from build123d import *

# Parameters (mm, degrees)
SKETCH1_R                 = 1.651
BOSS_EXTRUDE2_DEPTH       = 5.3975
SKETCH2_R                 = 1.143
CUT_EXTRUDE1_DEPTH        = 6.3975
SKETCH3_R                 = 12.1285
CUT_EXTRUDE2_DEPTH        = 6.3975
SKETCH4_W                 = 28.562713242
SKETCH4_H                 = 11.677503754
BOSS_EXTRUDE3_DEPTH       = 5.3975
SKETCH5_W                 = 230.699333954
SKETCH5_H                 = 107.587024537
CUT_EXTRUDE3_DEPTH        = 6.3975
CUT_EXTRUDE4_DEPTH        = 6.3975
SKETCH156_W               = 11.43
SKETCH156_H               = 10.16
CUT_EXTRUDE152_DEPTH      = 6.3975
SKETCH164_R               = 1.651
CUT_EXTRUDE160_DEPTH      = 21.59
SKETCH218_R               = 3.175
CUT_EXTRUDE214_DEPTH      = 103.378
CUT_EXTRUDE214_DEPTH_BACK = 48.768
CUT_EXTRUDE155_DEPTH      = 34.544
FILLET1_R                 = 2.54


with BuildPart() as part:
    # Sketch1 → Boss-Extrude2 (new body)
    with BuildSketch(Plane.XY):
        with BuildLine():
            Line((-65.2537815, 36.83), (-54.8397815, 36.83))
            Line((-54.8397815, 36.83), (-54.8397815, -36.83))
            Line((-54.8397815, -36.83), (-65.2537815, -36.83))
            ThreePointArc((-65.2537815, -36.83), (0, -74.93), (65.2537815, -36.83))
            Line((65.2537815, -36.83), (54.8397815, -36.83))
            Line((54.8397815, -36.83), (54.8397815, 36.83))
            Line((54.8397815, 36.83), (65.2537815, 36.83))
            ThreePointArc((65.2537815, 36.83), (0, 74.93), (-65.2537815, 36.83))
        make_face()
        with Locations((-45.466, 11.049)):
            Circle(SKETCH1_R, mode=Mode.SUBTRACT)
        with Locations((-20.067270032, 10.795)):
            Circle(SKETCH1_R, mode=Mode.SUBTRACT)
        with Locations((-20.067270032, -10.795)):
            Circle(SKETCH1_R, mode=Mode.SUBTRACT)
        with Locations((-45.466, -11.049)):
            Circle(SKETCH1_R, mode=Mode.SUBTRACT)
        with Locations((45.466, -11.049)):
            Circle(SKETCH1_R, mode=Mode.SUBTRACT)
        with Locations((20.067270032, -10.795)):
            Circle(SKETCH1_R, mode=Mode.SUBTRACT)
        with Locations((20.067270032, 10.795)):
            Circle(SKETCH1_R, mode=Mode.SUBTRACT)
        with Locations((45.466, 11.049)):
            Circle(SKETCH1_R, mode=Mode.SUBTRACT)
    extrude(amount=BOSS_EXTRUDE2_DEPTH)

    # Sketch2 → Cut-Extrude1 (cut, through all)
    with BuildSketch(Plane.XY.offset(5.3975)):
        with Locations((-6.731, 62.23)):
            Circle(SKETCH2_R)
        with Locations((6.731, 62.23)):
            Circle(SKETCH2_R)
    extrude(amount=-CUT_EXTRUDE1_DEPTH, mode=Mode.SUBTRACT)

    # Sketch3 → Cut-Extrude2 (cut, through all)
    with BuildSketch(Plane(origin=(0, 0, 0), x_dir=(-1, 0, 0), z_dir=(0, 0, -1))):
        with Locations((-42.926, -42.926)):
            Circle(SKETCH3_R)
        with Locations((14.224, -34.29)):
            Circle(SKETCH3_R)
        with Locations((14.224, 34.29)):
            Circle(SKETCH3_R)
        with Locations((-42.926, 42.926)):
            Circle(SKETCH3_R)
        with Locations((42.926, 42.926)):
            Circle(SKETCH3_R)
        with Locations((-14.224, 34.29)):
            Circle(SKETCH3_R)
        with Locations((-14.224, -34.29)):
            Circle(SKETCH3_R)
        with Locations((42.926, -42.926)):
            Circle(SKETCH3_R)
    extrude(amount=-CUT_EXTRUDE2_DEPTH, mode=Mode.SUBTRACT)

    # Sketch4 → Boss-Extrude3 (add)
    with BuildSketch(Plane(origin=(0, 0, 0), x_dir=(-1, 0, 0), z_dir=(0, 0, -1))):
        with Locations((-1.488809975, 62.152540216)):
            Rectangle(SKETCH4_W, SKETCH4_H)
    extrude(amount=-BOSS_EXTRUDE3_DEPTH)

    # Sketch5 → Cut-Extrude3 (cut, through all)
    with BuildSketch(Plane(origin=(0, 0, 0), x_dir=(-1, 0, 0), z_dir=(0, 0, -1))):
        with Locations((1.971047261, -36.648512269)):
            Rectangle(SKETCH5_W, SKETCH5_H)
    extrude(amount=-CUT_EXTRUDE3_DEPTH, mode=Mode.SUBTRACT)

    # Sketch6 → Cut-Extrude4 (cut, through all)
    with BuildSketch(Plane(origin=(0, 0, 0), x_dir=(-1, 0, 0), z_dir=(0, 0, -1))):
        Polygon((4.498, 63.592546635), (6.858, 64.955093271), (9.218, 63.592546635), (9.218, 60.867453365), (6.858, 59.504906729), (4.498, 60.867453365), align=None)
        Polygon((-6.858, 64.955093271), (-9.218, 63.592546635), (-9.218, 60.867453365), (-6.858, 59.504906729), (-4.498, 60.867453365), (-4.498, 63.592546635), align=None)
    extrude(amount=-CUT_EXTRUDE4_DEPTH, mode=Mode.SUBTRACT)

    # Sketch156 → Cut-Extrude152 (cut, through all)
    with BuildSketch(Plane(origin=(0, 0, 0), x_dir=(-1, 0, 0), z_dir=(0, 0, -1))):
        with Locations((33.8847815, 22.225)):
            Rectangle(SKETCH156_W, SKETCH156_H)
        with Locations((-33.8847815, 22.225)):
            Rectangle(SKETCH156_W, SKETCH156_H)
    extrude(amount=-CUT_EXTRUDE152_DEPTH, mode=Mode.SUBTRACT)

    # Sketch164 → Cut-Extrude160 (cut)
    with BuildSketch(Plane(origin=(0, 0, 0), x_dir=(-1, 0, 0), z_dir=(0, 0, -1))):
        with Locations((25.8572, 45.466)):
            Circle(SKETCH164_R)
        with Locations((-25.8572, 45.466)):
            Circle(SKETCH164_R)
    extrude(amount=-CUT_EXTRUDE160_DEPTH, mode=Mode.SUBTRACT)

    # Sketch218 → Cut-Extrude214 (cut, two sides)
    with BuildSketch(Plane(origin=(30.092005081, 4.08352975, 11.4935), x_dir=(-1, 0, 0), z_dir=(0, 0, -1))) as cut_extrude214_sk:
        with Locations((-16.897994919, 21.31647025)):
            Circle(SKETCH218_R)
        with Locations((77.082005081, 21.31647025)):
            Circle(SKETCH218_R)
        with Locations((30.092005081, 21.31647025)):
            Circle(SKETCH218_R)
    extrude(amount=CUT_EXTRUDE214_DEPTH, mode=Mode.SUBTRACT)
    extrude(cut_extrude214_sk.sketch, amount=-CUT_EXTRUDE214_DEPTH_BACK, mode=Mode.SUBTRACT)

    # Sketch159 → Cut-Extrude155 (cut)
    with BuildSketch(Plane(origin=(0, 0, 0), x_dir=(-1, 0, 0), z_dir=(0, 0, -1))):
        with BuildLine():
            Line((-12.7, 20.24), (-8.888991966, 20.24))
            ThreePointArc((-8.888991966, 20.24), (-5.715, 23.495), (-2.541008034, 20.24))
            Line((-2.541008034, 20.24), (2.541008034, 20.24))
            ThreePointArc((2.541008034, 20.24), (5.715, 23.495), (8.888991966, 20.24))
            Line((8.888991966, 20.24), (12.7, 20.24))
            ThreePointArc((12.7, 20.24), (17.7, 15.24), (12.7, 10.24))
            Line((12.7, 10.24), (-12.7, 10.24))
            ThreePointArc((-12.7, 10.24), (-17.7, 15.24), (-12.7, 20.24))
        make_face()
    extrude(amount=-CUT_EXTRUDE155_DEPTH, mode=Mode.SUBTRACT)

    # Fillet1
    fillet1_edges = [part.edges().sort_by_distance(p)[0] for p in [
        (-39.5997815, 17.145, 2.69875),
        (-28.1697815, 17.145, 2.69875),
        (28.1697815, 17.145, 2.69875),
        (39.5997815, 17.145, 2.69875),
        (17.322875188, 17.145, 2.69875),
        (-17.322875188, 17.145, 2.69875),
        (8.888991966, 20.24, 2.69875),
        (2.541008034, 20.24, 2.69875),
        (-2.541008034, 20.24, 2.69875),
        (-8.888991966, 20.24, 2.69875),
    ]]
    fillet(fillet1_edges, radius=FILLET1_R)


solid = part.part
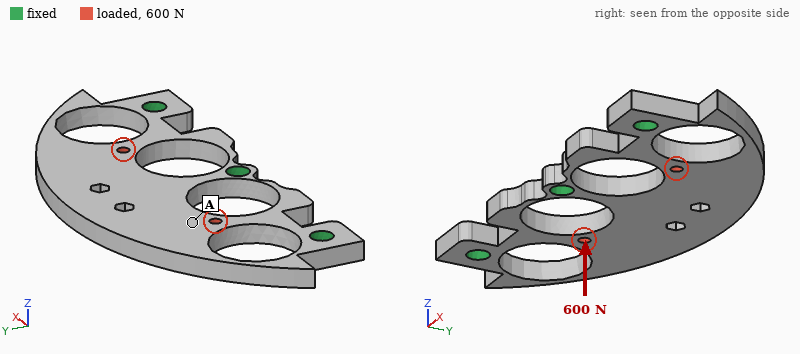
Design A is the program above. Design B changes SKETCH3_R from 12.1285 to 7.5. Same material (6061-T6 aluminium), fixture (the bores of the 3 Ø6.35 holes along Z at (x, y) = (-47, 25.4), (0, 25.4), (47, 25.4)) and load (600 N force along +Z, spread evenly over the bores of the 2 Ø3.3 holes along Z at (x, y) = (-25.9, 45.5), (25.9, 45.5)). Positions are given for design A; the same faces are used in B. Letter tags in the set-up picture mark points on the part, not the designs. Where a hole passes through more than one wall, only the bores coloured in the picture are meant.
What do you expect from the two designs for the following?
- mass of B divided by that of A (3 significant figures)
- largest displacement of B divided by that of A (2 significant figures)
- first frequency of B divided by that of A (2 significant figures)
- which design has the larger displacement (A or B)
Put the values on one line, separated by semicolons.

1.34; 0.38; 1.6; A
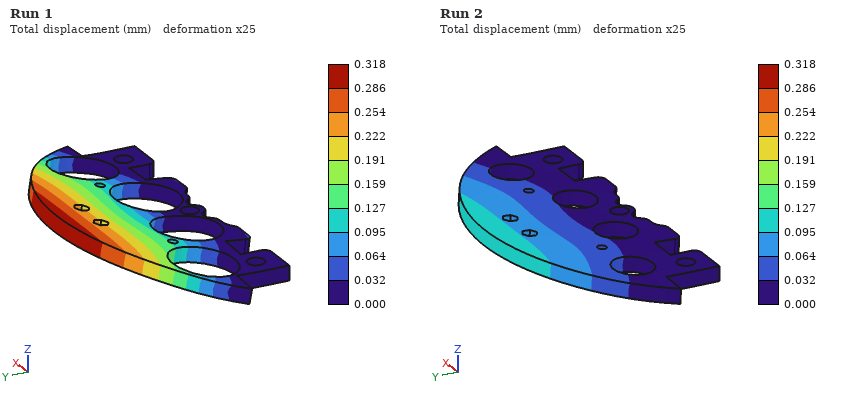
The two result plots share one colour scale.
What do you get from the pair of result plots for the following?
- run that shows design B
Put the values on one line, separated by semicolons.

Run 2
